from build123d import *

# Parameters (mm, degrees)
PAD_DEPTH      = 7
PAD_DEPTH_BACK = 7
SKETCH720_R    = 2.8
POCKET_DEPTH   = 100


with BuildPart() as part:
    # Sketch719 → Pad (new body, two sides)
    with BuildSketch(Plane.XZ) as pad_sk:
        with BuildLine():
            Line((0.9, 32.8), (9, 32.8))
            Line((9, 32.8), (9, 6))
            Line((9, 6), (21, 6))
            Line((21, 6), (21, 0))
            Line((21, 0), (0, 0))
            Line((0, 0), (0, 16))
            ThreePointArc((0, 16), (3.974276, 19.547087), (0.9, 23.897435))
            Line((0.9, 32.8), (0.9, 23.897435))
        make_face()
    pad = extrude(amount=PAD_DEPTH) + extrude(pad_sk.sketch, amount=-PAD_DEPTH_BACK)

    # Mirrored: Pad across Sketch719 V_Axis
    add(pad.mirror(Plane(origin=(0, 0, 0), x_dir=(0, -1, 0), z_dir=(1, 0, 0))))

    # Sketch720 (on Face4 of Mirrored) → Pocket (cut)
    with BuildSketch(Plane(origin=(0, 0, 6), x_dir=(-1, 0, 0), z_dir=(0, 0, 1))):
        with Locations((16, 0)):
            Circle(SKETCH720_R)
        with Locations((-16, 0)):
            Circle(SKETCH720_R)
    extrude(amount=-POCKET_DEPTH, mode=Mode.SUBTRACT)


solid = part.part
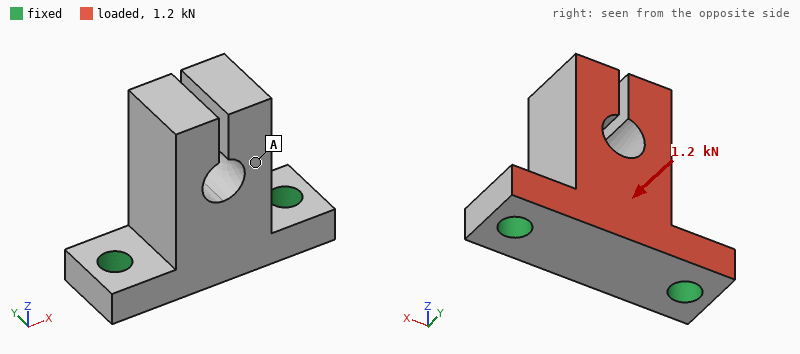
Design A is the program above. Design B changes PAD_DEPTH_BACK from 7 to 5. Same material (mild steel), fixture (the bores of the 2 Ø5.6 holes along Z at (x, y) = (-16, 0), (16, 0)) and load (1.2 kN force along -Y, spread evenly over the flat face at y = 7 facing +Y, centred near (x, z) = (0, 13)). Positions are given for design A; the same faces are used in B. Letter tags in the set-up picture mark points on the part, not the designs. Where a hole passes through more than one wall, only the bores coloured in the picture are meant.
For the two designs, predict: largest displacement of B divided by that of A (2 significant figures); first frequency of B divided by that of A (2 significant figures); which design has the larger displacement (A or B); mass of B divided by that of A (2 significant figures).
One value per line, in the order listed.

1.3
0.95
B
0.85
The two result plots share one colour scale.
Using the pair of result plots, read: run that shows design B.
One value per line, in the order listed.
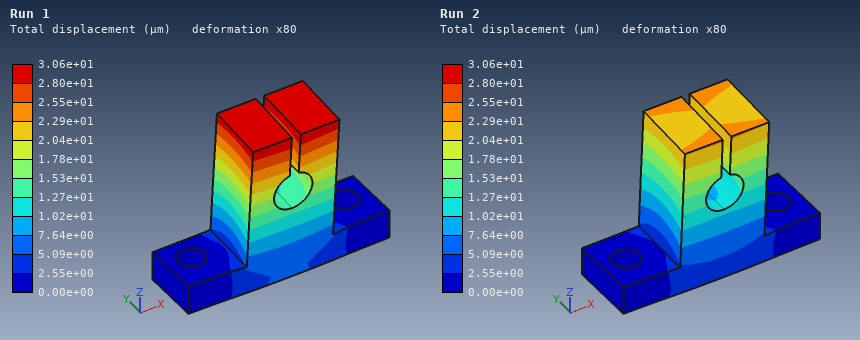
Run 1
